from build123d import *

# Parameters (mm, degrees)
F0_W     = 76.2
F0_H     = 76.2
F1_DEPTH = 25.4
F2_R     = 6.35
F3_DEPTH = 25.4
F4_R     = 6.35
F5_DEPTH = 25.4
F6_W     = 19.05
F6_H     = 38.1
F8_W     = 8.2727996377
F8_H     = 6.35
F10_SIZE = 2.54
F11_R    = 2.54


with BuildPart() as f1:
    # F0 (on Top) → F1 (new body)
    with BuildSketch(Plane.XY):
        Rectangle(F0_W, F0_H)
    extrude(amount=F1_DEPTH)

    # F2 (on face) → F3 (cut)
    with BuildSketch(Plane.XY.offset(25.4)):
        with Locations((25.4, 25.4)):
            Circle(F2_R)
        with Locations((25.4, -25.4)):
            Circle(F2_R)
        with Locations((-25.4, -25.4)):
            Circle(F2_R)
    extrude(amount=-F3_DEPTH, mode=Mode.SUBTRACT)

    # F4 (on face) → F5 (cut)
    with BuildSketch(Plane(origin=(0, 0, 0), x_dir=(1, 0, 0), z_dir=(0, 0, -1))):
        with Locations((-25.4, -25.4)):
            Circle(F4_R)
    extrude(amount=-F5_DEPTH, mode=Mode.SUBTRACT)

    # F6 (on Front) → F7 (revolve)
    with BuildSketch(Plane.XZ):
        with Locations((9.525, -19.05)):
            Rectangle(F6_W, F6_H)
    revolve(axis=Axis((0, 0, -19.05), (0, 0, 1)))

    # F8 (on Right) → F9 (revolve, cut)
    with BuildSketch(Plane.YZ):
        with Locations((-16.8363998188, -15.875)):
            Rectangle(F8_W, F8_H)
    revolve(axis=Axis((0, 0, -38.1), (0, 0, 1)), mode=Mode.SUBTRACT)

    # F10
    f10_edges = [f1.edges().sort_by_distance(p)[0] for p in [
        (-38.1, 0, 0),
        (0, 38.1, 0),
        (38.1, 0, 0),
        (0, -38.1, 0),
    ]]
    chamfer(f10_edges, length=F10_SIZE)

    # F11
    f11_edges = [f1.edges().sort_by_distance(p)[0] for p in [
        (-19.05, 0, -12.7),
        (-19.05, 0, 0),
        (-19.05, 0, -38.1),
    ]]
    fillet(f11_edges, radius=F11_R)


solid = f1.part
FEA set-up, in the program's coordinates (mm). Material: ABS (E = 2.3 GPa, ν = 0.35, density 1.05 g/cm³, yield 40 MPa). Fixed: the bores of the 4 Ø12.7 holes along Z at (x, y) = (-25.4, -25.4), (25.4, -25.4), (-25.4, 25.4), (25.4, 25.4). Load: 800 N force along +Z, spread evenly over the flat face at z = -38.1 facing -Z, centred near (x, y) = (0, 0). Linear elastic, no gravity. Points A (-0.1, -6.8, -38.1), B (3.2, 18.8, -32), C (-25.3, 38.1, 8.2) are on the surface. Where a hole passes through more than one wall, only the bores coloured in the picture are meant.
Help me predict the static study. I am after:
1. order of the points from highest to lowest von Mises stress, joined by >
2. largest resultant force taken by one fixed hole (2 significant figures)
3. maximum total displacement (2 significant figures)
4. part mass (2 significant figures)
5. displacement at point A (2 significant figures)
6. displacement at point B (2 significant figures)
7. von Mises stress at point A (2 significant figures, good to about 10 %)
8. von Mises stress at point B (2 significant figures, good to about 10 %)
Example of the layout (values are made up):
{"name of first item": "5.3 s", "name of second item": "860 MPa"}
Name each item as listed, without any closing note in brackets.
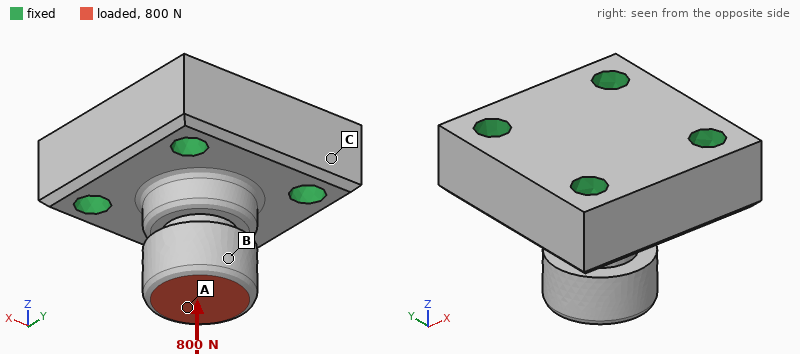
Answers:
{"order of the points from highest to lowest von Mises stress, joined by >": "A > B > C", "largest resultant force taken by one fixed hole": "210 N", "maximum total displacement": "26 µm", "part mass": "180 g", "displacement at point A": "26 µm", "displacement at point B": "24 µm", "von Mises stress at point A": "0.90 MPa", "von Mises stress at point B": "0.38 MPa"}
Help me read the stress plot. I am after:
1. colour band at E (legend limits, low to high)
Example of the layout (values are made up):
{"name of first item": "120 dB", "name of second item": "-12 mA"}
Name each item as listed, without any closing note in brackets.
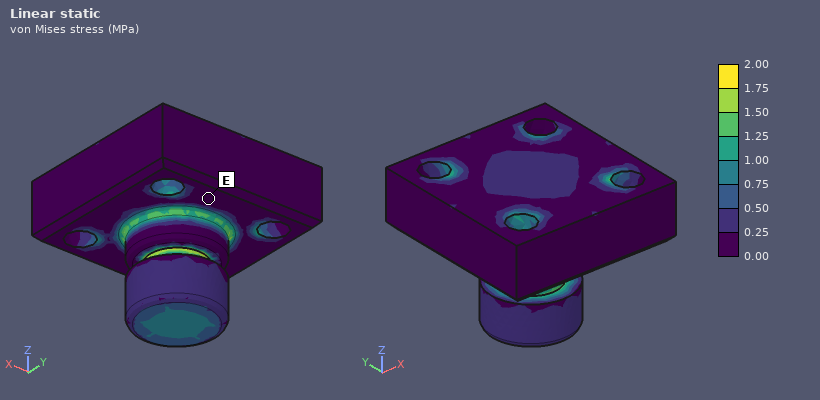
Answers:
{"colour band at E": "0.00 to 0.25 MPa"}
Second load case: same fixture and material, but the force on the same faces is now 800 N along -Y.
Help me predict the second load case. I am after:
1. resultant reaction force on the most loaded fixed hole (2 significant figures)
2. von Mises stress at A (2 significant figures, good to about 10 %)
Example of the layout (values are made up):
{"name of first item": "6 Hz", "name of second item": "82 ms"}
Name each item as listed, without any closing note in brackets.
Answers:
{"resultant reaction force on the most loaded fixed hole": "470 N", "von Mises stress at A": "1.9 MPa"}
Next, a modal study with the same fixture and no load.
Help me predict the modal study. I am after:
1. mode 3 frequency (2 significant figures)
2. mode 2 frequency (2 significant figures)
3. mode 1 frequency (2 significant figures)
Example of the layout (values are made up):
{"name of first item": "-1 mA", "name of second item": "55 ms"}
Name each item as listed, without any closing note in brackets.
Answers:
{"mode 3 frequency": "3700 Hz", "mode 2 frequency": "2400 Hz", "mode 1 frequency": "2400 Hz"}
